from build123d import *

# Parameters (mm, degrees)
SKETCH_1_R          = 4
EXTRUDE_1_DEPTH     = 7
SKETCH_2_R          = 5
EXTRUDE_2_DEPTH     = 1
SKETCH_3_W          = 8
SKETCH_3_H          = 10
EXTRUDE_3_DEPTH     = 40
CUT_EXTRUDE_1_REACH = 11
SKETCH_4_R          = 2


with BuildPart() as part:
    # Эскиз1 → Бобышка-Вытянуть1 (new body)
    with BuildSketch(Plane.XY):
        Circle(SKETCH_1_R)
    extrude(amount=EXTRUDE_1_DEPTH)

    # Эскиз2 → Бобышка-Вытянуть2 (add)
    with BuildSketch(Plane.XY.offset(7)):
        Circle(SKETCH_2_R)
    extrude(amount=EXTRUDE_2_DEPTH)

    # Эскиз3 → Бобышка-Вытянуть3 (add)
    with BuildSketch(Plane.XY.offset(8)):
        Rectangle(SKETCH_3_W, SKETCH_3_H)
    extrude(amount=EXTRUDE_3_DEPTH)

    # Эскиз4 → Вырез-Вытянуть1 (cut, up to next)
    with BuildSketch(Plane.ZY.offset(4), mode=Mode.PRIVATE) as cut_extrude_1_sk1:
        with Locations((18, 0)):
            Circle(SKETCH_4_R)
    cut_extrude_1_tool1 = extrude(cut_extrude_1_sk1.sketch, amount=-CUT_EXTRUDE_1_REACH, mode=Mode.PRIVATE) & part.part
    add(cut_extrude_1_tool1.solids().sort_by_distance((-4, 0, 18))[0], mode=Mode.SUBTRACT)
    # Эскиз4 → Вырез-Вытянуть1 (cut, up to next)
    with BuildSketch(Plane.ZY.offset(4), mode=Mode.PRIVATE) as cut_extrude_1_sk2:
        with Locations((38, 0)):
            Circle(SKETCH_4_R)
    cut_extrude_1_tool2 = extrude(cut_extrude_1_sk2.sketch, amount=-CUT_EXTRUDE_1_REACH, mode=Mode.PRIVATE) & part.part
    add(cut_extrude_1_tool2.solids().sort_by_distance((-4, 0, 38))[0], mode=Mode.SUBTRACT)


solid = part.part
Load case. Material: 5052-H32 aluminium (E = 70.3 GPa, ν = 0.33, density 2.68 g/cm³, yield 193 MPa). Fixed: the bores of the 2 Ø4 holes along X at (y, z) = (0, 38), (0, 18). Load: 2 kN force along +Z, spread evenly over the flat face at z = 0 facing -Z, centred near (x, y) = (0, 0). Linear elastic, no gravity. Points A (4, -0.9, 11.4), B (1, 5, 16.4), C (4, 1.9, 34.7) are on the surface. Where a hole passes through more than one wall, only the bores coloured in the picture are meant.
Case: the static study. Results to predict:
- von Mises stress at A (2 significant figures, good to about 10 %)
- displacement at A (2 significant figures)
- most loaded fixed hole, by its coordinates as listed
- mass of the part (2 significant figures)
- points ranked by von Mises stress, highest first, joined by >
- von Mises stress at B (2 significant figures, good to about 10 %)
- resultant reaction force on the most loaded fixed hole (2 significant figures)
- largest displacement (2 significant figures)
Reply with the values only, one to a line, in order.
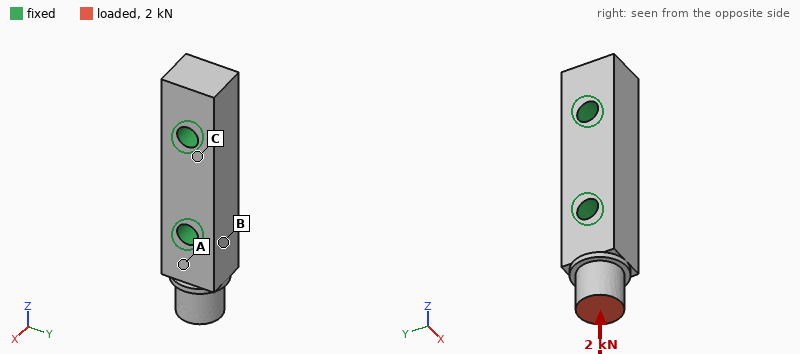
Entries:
33 MPa
2.4 µm
(0, 18)
9.2 g
A > B > C
13 MPa
1.9 kN
8.2 µm
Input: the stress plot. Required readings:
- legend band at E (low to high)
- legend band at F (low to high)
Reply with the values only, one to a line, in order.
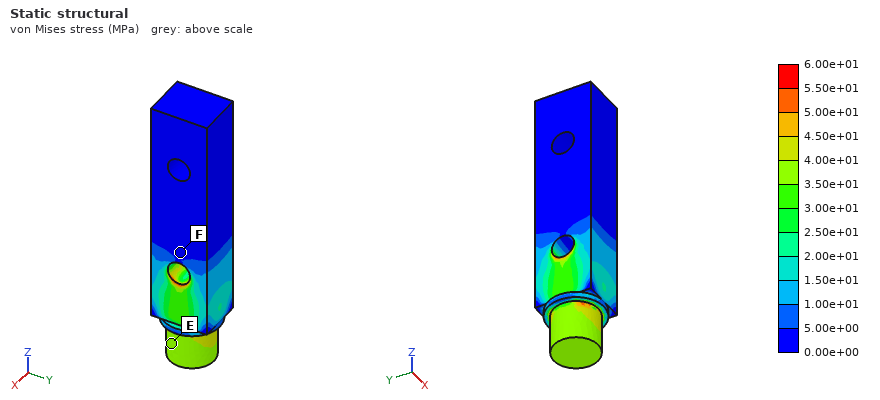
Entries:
3.50e+01 to 4.00e+01 MPa
0.00e+00 to 5.00e+00 MPa
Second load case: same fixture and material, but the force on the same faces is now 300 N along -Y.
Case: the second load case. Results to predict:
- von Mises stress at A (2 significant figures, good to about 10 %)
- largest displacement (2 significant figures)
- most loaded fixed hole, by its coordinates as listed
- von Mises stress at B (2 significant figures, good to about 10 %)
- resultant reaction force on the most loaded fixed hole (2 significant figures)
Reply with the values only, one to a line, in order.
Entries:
10 MPa
23 µm
(0, 18)
30 MPa
390 N
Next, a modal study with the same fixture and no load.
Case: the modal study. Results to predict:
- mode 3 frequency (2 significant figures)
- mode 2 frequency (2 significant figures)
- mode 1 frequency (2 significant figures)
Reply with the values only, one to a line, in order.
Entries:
48 kHz
23 kHz
22 kHz
